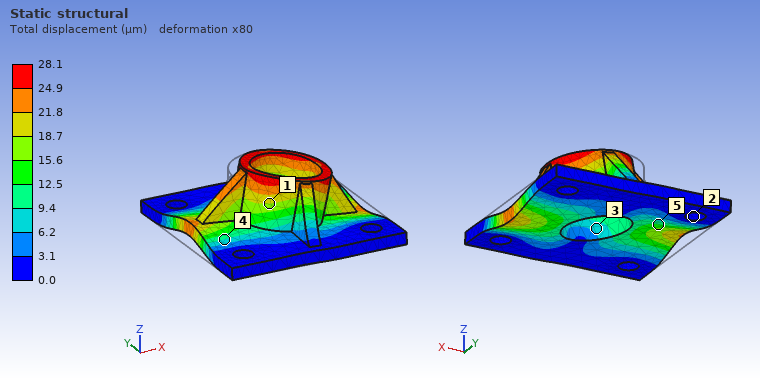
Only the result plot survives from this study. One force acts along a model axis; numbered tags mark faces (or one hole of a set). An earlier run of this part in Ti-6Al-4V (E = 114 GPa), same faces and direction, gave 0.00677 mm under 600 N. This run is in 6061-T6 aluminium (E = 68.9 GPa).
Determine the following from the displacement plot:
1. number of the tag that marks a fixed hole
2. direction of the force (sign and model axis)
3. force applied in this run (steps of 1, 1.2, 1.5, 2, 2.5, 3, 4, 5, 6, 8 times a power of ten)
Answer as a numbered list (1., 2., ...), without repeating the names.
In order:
1. 2
2. +X
3. 1.5 kN
